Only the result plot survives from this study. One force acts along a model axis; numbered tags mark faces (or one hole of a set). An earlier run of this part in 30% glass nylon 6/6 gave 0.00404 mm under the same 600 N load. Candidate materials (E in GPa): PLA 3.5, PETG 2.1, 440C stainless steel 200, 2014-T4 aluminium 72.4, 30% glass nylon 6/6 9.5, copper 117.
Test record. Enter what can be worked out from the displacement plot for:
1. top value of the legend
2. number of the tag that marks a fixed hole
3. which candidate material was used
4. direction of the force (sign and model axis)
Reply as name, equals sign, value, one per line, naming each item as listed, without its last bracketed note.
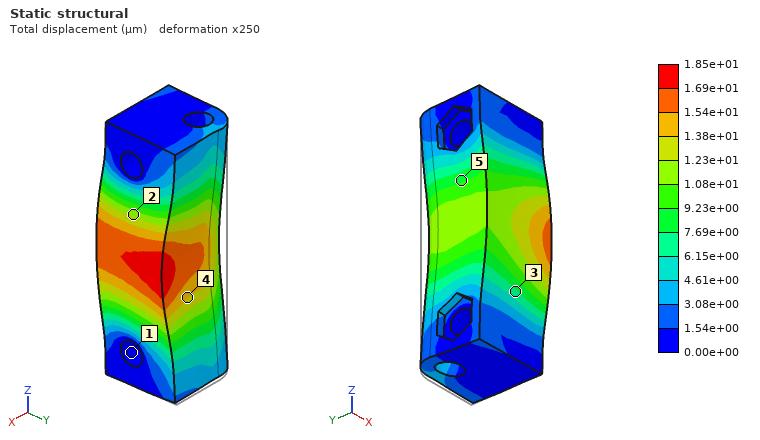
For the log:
top value of the legend = 1.85e+01 µm
number of the tag that marks a fixed hole = 1
which candidate material was used = PETG
direction of the force = -Y
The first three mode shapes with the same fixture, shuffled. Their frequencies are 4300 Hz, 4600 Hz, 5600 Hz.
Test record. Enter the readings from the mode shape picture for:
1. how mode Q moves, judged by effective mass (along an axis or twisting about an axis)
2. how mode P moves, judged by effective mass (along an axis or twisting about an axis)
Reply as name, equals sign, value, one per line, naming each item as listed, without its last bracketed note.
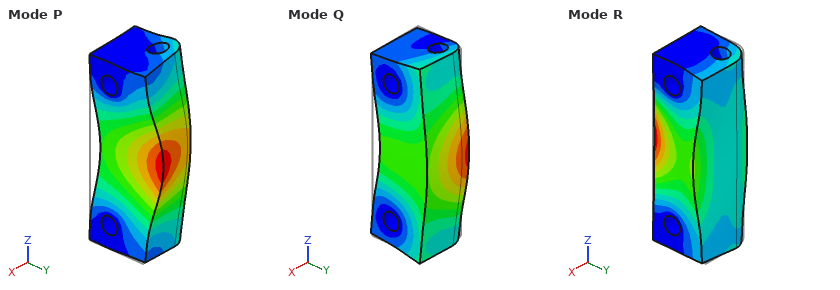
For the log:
how mode Q moves, judged by effective mass = along Y
how mode P moves, judged by effective mass = along X
